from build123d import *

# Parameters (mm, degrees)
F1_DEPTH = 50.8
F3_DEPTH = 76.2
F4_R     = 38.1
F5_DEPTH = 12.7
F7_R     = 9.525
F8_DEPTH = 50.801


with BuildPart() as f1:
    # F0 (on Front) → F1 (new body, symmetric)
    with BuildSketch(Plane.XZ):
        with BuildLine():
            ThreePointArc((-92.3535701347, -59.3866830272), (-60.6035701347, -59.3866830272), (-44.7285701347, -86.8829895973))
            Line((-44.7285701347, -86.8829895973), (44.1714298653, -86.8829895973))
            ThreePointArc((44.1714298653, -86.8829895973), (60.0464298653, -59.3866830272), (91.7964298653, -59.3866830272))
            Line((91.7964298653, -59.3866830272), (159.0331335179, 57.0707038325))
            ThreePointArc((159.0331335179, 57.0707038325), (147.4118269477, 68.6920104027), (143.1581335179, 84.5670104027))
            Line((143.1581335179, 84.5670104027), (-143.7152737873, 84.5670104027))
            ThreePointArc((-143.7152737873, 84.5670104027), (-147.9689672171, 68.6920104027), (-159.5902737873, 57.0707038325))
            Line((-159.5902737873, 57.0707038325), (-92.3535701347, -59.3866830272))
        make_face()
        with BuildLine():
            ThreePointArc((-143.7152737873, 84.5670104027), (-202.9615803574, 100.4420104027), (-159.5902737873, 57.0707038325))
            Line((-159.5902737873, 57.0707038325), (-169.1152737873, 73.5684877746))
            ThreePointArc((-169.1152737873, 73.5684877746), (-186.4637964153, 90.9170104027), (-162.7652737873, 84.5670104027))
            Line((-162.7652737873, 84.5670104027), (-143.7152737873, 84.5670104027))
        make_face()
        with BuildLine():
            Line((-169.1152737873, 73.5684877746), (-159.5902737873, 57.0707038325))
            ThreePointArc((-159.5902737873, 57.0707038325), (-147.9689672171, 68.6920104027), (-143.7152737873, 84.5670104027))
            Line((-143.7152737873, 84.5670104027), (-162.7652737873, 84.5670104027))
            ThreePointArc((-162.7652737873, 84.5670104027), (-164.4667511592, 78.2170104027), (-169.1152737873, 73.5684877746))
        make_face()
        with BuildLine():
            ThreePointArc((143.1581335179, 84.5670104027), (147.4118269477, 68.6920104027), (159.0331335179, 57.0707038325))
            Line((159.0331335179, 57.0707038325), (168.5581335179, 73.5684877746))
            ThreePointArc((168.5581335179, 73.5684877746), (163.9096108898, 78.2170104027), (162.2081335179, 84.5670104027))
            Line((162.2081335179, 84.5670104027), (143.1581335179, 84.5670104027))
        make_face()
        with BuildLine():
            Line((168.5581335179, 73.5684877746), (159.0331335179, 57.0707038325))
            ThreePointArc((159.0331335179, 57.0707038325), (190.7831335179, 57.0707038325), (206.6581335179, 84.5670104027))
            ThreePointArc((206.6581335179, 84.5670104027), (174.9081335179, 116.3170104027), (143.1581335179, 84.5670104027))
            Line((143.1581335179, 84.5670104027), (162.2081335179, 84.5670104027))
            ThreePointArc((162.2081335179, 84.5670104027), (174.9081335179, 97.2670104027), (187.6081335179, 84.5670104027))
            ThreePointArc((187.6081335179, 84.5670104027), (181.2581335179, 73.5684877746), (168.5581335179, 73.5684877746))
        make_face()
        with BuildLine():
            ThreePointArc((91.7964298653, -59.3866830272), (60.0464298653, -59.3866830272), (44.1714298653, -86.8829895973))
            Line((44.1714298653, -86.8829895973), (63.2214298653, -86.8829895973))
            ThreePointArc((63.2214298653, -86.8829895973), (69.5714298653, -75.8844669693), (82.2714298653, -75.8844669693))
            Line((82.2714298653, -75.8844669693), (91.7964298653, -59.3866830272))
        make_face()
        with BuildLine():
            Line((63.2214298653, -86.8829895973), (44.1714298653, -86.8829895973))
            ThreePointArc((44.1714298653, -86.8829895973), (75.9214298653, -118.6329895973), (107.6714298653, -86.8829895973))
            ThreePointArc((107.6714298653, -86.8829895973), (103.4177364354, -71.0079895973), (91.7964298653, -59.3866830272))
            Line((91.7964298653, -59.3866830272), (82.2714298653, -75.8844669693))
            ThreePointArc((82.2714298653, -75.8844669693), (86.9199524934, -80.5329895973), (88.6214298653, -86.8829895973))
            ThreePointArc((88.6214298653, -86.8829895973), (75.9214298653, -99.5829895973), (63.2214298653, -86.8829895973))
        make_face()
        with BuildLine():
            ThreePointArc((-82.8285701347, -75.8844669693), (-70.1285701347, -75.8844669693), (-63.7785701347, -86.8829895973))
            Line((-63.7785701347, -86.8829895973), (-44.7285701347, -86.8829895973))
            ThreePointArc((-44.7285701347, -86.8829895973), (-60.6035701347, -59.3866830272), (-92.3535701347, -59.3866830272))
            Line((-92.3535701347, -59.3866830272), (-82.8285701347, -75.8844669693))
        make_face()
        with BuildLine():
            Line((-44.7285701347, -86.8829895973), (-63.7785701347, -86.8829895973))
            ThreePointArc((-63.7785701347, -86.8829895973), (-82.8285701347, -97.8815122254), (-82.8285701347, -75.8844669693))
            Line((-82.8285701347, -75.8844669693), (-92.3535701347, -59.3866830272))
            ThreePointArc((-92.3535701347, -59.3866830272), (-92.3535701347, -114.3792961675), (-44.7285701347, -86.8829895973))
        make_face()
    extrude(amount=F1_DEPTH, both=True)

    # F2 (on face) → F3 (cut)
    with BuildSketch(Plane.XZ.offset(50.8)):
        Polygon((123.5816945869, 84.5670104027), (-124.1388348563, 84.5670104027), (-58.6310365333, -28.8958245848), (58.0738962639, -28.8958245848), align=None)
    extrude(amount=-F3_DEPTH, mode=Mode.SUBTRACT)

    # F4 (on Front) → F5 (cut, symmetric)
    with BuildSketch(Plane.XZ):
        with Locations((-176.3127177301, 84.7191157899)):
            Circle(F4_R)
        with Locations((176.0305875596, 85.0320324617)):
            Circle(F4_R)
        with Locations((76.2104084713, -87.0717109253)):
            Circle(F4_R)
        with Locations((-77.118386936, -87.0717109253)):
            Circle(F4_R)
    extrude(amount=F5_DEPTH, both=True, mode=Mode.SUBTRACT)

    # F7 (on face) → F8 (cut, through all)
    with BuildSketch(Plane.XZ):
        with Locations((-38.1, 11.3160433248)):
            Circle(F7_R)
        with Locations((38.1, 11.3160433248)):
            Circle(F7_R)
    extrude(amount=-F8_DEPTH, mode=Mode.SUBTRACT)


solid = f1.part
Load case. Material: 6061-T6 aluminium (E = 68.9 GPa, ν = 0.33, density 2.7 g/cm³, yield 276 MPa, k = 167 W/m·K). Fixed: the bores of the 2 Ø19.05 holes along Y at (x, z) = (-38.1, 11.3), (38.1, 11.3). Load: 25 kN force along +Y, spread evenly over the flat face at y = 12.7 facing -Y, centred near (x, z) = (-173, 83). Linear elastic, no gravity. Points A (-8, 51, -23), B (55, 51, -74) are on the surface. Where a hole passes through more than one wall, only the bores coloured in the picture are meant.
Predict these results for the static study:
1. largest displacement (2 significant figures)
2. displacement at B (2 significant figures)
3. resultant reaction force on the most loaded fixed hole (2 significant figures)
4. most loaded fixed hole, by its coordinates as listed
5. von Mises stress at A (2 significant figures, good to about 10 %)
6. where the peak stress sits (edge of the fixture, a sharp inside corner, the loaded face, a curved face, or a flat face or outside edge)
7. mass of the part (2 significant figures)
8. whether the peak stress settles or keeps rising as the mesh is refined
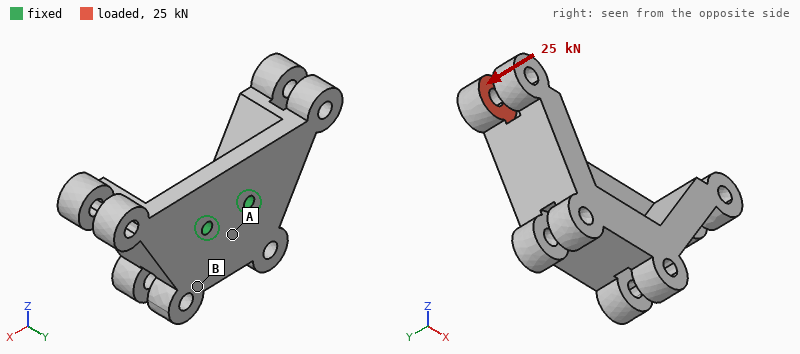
1.1 mm
0.25 mm
51 kN
(-38.1, 11.3)
41 MPa
edge of the fixture
8.8 kg
keeps rising
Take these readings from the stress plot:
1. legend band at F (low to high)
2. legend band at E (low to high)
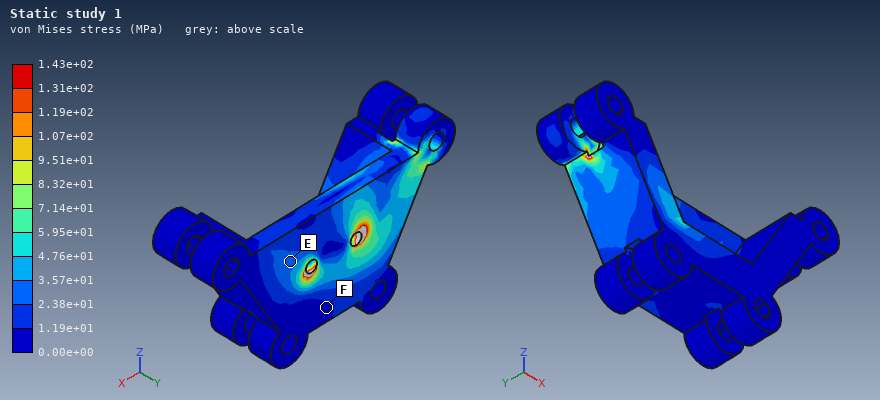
0.00e+00 to 1.19e+01 MPa
2.38e+01 to 3.57e+01 MPa
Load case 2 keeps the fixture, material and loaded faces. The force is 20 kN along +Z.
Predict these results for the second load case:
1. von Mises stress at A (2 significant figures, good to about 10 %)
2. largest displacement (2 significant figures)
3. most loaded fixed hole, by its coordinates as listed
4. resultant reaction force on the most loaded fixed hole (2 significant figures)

19 MPa
0.41 mm
(-38.1, 11.3)
48 kN
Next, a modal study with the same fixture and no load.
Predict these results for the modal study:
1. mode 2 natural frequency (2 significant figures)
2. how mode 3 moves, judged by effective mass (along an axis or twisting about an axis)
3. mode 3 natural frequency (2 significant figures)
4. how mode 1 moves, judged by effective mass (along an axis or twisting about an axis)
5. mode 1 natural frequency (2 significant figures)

790 Hz
twisting about Y
1200 Hz
along Z
640 Hz
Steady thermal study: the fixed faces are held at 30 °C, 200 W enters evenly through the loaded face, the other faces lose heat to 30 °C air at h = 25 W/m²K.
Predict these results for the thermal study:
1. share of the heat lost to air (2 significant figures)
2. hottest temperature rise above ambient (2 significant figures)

30 %
67 K
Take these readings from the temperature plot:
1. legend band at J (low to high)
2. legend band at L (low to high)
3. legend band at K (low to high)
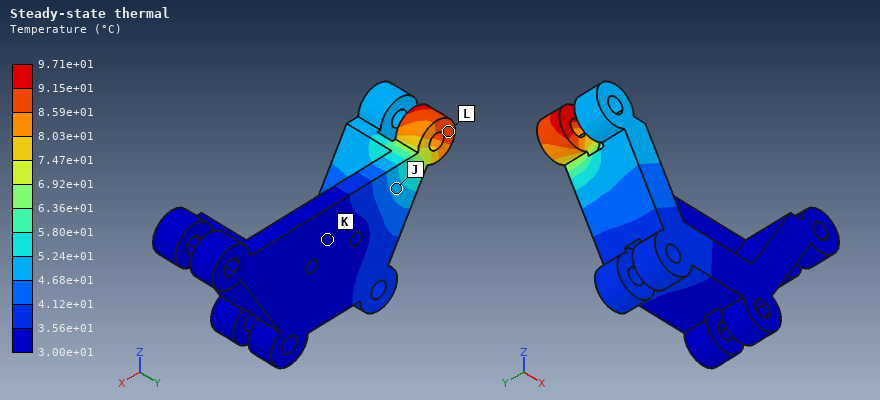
4.68e+01 to 5.24e+01 °C
8.59e+01 to 9.15e+01 °C
3.00e+01 to 3.56e+01 °C
